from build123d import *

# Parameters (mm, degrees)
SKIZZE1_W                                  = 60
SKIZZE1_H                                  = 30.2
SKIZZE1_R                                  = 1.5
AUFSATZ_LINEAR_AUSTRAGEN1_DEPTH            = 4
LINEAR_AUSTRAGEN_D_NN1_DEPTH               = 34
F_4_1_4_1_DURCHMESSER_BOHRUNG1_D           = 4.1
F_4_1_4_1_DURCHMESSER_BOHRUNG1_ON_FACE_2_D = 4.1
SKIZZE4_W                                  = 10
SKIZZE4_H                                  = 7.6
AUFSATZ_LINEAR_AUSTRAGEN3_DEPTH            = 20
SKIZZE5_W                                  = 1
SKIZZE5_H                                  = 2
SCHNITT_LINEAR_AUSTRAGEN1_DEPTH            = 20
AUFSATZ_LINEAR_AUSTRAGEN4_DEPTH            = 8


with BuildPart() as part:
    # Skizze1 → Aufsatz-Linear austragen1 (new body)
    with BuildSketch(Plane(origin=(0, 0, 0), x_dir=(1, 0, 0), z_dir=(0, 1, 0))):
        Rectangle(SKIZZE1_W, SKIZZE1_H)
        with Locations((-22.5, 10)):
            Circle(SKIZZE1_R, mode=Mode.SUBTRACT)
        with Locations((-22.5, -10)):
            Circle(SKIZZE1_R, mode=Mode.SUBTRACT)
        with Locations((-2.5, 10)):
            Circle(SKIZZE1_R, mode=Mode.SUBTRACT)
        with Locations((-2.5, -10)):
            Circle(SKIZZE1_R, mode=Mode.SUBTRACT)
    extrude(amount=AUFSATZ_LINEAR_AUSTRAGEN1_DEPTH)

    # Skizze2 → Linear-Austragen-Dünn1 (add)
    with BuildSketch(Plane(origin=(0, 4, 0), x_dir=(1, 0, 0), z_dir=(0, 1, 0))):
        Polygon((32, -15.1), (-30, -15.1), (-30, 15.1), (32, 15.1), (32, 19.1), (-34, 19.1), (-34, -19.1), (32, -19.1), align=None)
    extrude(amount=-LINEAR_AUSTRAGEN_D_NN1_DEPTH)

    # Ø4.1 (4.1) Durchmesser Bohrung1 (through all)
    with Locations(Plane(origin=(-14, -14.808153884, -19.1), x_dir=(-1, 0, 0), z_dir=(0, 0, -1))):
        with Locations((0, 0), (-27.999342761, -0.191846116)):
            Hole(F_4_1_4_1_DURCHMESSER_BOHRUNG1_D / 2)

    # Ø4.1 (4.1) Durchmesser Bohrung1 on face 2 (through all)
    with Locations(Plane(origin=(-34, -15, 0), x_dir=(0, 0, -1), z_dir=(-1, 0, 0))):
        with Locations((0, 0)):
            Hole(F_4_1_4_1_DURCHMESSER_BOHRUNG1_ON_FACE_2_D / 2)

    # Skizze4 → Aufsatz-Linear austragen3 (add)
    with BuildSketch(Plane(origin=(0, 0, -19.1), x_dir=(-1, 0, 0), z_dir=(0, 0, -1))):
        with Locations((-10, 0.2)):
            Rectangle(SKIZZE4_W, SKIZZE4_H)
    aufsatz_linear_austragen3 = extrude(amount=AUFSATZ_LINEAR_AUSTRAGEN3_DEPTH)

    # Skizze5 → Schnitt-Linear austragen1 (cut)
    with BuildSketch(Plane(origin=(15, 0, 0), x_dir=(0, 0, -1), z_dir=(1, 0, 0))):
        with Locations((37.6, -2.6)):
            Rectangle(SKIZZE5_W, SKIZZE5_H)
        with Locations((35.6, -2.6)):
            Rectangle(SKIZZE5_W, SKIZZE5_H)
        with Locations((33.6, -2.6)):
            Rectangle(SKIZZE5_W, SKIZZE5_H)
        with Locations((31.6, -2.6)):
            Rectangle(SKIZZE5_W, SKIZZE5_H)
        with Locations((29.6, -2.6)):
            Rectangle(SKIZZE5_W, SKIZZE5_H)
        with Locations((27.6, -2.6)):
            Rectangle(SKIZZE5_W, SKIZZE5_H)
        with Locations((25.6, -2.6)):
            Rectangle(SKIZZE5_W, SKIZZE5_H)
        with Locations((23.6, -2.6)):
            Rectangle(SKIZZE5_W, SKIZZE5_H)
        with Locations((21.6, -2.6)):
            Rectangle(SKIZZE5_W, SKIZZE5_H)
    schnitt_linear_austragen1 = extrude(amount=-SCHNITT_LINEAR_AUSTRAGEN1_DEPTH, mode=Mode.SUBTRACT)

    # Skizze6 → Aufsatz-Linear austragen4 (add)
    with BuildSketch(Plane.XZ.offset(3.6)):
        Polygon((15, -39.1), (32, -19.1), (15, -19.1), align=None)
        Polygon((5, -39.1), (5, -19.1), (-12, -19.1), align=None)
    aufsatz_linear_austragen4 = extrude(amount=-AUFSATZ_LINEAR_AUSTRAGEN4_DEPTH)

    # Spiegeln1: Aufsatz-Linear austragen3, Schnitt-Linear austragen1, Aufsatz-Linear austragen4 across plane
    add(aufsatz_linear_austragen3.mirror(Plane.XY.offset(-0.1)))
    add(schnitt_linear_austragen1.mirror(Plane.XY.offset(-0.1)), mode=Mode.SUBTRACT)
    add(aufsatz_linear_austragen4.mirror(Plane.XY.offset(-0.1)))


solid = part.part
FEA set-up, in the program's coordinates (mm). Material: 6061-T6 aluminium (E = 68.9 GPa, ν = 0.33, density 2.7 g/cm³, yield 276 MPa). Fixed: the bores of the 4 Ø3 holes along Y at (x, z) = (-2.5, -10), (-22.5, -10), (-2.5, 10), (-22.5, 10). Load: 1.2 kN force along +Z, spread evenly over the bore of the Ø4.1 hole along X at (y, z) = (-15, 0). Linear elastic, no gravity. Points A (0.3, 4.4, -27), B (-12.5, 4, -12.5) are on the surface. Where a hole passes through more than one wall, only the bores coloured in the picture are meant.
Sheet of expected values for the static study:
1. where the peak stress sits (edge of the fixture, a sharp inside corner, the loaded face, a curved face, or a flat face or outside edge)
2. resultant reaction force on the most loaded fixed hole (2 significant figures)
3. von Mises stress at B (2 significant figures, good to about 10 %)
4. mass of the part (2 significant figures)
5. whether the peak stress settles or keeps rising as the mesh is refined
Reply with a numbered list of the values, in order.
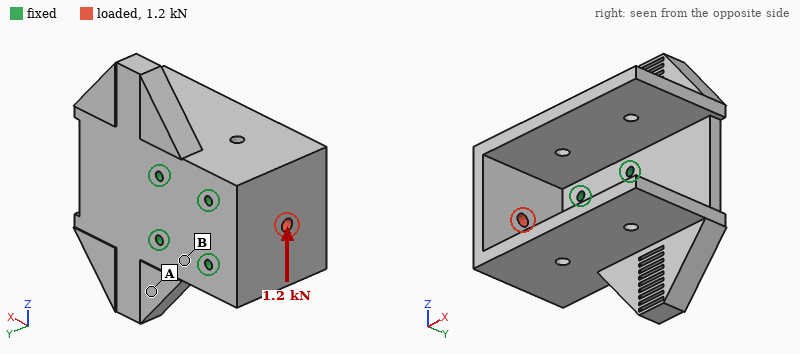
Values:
1. edge of the fixture
2. 1.0 kN
3. 14 MPa
4. 100 g
5. keeps rising
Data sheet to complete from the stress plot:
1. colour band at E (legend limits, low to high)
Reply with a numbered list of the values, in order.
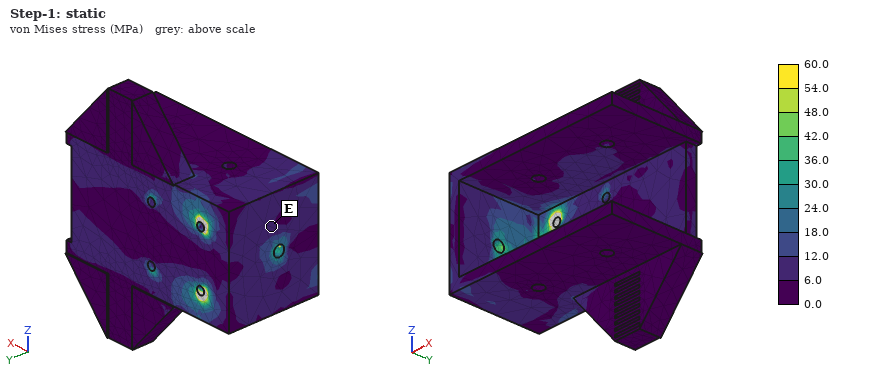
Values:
1. 6.0 to 12.0 MPa
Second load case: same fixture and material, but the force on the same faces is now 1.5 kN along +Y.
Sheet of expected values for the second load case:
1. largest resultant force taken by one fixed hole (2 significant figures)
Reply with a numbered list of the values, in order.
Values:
1. 970 N
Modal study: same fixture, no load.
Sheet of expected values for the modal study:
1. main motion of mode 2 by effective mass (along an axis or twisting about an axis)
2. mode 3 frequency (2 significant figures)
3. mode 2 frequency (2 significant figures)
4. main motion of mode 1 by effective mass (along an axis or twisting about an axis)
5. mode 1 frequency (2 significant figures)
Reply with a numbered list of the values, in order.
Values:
1. along Z
2. 4100 Hz
3. 2600 Hz
4. along Y
5. 2500 Hz
